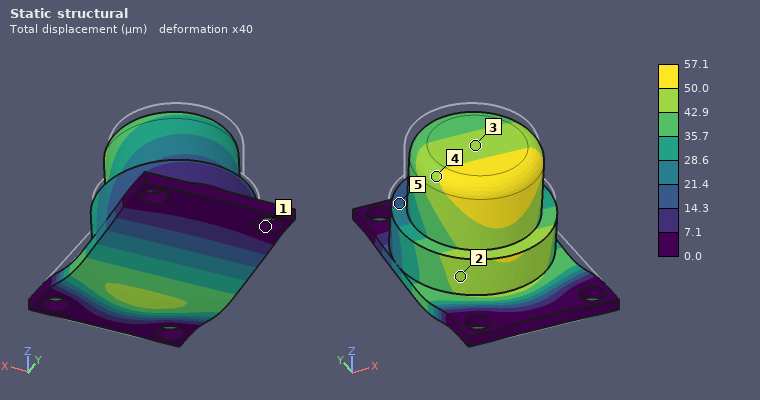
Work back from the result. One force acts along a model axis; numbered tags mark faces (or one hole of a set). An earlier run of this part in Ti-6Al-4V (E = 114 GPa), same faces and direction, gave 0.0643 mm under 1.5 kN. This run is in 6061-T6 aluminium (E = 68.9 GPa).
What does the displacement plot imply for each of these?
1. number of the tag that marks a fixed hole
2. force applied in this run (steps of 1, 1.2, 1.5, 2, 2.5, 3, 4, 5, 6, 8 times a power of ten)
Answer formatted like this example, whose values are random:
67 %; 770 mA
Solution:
1; 800 N
